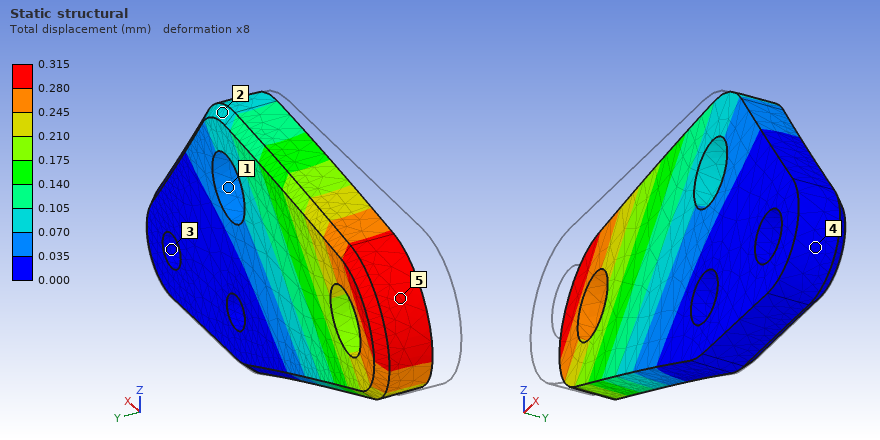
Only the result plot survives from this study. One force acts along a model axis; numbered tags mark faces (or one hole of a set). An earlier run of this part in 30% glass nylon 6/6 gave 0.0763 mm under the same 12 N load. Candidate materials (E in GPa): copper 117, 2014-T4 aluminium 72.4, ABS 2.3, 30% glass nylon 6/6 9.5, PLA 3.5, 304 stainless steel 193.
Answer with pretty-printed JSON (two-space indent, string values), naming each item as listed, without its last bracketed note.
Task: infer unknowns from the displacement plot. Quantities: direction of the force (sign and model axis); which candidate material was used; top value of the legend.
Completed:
{
  "direction of the force": "+Y",
  "which candidate material was used": "ABS",
  "top value of the legend": "0.315 mm"
}
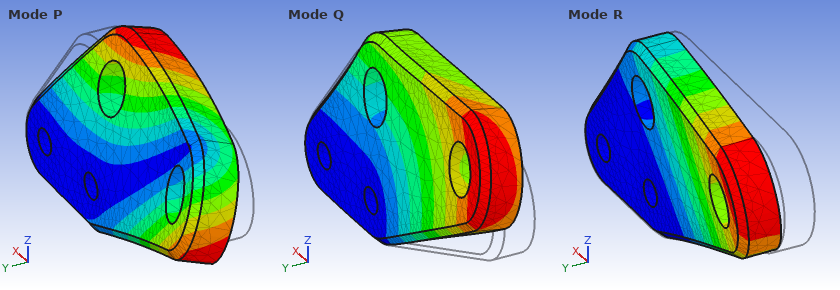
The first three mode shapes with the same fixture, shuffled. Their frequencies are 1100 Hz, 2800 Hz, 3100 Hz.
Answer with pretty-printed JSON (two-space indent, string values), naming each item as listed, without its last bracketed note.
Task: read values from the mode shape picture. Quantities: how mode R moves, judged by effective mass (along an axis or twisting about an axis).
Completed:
{
  "how mode R moves, judged by effective mass": "along Y"
}
